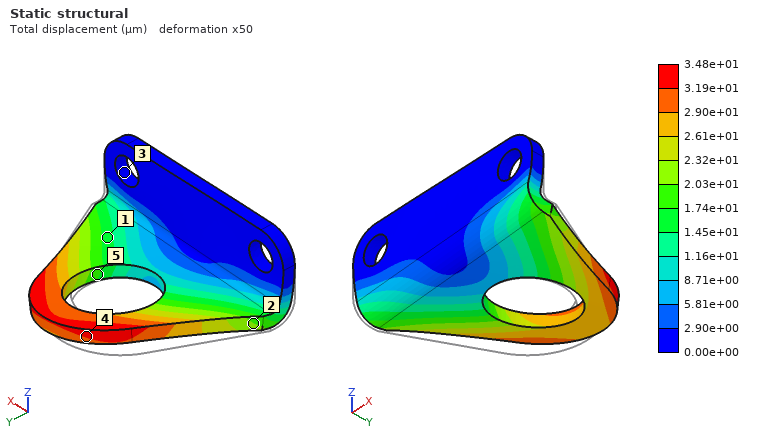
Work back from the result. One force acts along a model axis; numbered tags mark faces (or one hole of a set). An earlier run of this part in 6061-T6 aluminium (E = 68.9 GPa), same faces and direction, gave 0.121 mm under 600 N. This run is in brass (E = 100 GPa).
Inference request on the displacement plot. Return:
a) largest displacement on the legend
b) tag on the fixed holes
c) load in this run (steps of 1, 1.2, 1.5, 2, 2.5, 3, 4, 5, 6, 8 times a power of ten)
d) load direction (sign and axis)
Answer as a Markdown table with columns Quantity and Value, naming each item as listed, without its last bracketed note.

| Quantity | Value |
|---|---|
| largest displacement on the legend | 3.48e+01 µm |
| tag on the fixed holes | 3 |
| load in this run | 250 N |
| load direction | +X |
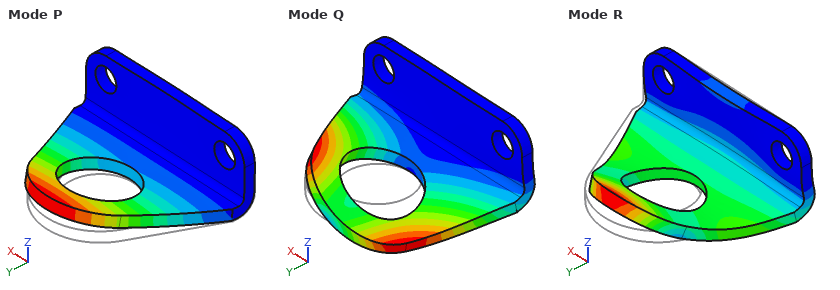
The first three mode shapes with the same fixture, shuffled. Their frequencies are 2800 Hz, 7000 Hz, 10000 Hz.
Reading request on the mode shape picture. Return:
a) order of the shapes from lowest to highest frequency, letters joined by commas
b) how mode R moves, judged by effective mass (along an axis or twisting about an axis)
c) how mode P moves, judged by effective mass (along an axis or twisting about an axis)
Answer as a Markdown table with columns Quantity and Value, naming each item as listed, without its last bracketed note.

| Quantity | Value |
|---|---|
| order of the shapes from lowest to highest frequency, letters joined by commas | P, Q, R |
| how mode R moves, judged by effective mass | along Y |
| how mode P moves, judged by effective mass | along Z |
